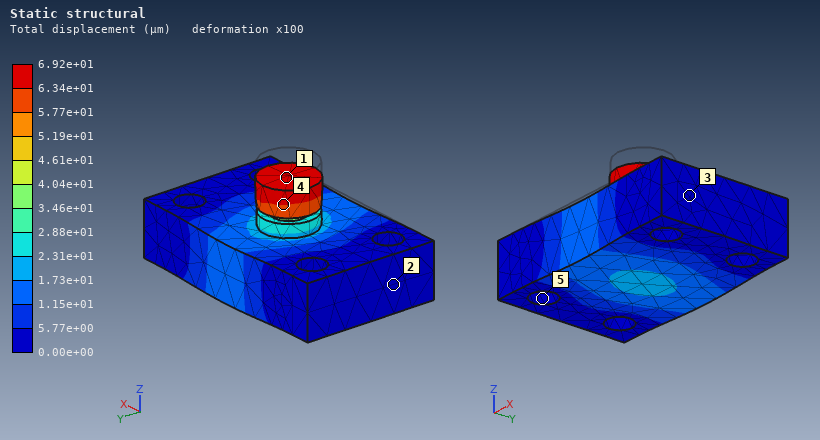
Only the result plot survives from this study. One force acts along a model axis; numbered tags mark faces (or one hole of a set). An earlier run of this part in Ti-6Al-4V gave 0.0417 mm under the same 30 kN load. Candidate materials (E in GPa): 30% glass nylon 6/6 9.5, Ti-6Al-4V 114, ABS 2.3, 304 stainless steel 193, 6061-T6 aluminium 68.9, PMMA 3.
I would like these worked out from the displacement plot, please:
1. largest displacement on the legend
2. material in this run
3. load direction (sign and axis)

6.92e+01 µm
6061-T6 aluminium
-Z
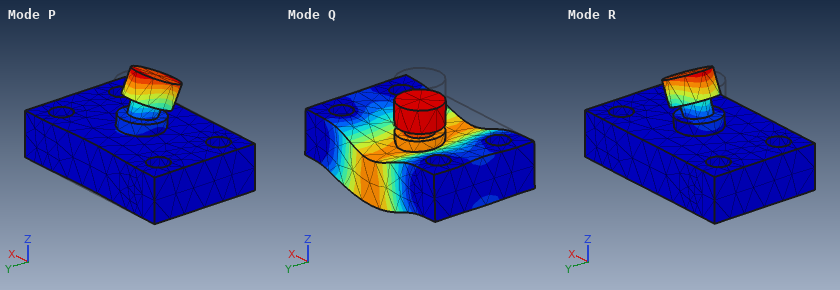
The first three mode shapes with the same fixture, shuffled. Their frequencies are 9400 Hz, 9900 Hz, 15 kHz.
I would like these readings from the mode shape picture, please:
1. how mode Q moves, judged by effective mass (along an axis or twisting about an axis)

along Z
